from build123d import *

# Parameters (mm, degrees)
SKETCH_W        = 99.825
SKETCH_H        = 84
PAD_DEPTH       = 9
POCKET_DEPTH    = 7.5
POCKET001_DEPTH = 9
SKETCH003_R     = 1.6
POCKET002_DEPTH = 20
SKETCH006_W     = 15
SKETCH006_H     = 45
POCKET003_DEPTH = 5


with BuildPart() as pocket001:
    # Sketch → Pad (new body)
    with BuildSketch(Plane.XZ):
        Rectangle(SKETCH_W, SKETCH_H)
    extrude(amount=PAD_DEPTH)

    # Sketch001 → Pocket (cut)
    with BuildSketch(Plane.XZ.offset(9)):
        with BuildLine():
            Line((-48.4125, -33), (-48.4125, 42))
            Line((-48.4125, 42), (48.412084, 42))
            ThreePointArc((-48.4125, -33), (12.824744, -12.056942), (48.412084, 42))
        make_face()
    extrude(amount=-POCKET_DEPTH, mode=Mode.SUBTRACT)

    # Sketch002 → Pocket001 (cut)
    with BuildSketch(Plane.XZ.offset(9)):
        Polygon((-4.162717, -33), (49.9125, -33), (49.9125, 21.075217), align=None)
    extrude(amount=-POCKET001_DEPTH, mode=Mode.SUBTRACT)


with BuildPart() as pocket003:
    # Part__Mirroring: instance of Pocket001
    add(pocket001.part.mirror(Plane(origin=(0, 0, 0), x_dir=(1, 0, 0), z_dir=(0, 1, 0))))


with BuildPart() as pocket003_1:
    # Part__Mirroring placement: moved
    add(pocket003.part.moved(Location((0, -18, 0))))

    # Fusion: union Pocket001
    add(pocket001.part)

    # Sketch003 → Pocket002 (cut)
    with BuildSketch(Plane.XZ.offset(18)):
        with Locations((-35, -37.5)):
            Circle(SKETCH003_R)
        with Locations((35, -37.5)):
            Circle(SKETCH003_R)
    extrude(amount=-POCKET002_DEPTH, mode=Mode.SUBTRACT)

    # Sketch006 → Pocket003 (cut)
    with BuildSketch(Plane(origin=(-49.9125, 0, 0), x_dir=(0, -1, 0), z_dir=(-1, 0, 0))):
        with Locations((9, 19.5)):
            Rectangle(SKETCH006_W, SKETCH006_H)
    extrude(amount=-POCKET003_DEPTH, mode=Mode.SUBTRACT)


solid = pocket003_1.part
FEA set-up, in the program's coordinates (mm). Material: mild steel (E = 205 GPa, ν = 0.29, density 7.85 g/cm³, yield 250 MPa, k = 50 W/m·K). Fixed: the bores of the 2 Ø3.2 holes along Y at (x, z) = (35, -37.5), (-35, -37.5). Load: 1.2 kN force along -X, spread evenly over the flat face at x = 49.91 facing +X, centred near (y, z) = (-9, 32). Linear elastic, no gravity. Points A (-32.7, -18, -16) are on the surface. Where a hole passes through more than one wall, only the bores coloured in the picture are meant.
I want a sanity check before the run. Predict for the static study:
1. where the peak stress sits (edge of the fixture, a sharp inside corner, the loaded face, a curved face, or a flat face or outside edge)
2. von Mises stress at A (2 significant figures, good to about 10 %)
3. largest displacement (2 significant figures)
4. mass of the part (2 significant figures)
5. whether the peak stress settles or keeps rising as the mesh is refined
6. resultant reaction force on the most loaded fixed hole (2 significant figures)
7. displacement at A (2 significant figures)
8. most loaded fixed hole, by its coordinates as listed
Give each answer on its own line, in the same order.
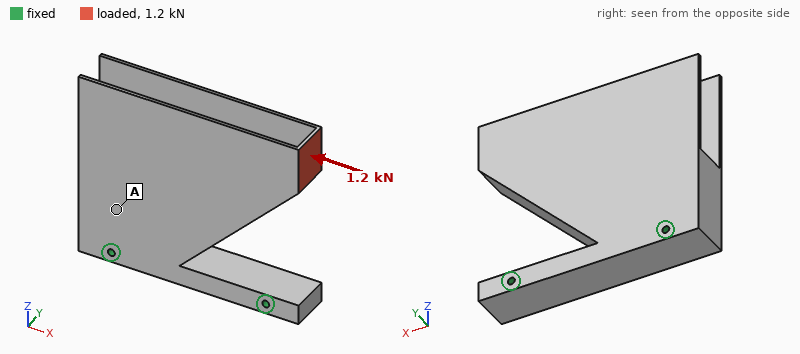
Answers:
edge of the fixture
22 MPa
0.13 mm
330 g
keeps rising
1.2 kN
0.019 mm
(-35, -37.5)
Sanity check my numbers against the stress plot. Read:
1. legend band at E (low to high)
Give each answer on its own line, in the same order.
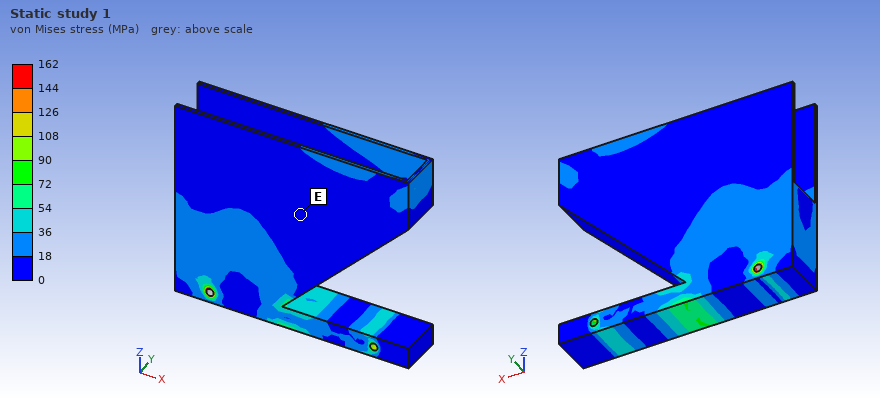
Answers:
0 to 18 MPa
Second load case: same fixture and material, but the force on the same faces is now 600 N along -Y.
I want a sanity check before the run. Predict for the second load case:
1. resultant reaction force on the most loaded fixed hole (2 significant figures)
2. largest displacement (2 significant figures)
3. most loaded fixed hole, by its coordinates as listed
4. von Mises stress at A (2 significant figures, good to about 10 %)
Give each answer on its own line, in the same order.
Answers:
520 N
0.37 mm
(35, -37.5)
30 MPa
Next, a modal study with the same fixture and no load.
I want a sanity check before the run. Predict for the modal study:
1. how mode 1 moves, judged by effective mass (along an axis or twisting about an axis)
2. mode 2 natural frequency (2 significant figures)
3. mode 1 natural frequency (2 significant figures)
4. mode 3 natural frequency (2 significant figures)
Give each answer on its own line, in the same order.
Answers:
along Y
570 Hz
530 Hz
990 Hz
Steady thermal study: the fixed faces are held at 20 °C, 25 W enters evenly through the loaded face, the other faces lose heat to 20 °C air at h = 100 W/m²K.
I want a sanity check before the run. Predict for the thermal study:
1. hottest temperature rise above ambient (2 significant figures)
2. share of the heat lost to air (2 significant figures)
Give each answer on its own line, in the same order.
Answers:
83 K
98 %
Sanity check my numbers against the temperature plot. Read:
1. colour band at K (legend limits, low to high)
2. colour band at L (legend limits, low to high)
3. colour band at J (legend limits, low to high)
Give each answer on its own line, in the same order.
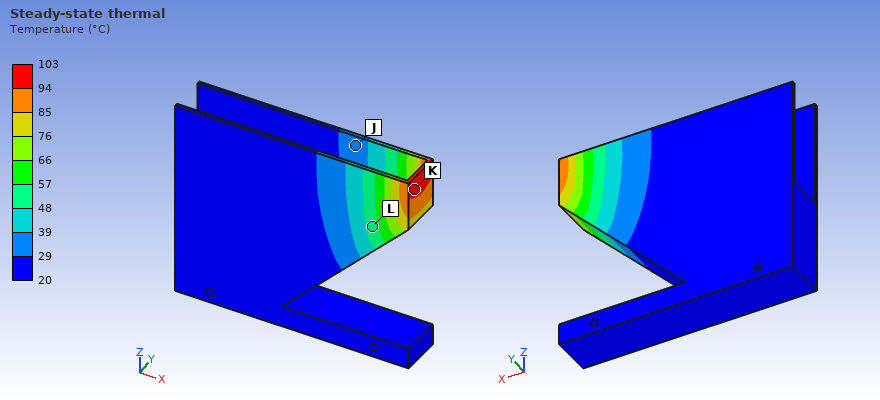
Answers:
94 to 103 °C
48 to 57 °C
29 to 39 °C
